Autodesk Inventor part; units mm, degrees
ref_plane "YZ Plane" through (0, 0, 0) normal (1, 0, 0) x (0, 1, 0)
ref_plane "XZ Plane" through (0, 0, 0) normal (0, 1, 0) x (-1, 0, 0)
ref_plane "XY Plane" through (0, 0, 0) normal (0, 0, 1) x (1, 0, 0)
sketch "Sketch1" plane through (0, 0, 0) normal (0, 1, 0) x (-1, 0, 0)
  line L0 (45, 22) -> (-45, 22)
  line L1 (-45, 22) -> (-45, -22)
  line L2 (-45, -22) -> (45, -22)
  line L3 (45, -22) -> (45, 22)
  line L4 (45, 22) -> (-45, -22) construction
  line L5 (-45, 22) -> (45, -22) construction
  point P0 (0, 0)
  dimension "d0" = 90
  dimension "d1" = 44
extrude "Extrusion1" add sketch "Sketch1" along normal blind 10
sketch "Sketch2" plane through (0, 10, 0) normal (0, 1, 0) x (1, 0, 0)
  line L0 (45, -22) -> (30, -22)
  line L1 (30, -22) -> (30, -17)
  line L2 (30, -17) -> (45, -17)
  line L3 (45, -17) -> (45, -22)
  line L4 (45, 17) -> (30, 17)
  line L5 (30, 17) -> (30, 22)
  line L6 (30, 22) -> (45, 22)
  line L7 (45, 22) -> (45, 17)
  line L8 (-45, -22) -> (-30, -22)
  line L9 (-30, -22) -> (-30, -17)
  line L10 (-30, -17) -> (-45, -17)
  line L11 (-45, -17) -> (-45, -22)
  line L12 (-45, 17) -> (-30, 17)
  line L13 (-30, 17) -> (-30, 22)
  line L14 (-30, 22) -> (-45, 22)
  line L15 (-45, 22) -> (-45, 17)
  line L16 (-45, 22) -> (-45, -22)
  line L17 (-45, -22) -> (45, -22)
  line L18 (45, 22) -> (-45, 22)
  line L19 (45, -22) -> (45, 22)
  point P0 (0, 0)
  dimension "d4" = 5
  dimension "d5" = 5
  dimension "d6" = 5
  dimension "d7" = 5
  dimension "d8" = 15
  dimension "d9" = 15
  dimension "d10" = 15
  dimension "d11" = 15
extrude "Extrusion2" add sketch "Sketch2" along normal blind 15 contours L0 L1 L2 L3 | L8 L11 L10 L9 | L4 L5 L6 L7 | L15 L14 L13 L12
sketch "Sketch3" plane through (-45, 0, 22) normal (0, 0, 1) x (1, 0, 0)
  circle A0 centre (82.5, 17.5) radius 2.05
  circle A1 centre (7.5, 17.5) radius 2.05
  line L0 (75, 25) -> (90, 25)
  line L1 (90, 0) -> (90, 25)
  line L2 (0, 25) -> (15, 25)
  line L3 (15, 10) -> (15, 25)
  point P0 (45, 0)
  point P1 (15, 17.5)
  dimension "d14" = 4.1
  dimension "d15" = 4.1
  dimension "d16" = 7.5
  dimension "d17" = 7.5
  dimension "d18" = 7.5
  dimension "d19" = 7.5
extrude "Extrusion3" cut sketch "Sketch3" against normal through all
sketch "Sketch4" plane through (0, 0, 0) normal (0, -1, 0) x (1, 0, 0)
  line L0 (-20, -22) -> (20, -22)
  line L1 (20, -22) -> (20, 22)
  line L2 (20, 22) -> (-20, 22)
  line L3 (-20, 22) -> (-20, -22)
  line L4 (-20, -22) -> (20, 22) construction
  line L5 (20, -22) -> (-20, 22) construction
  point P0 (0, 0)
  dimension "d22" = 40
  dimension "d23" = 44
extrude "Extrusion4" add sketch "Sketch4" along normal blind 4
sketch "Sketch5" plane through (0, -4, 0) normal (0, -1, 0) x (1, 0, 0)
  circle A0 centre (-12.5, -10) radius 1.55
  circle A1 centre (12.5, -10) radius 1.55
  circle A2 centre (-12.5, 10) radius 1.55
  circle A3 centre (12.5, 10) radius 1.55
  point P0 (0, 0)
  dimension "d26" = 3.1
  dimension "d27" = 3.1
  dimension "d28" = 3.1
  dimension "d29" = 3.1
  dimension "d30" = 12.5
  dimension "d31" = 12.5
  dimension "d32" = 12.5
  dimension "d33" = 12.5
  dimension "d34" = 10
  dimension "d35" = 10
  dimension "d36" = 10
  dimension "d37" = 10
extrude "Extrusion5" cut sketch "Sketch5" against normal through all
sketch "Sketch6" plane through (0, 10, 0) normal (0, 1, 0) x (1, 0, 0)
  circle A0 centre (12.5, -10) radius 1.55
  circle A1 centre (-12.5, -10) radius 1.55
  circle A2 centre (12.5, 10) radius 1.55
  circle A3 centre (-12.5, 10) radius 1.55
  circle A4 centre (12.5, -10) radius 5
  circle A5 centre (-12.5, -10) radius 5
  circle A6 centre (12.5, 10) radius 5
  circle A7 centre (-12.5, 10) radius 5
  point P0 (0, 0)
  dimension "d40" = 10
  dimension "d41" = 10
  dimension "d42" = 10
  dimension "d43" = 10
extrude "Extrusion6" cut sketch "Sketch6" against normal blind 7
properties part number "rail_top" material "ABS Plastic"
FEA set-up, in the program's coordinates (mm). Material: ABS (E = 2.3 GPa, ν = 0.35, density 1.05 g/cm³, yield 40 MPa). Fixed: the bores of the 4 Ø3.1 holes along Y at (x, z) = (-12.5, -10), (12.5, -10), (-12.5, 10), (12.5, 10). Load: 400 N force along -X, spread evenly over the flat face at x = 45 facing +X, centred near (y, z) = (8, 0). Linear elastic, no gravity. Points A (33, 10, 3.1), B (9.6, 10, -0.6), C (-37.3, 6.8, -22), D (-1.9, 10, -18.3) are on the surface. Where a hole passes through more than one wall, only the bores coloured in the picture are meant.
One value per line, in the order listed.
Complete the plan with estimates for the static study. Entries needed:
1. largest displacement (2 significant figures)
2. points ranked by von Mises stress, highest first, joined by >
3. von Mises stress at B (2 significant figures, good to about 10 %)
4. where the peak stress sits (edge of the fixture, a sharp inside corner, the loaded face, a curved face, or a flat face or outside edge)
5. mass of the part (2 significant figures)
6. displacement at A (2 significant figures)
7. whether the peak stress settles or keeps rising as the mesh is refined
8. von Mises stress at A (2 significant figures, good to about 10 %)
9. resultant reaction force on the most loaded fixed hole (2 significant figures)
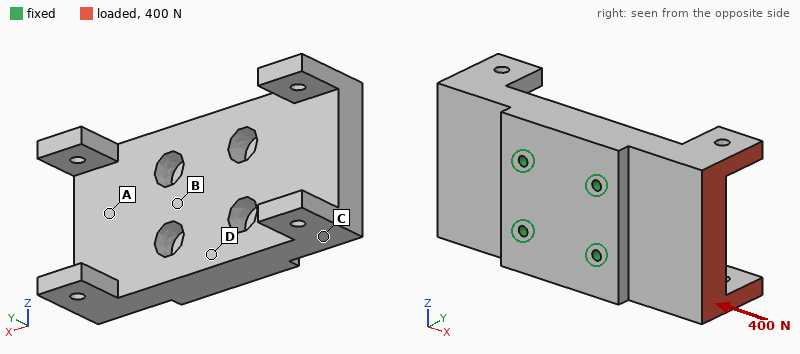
0.21 mm
B > A > D > C
2.3 MPa
edge of the fixture
51 g
0.076 mm
keeps rising
1.6 MPa
120 N
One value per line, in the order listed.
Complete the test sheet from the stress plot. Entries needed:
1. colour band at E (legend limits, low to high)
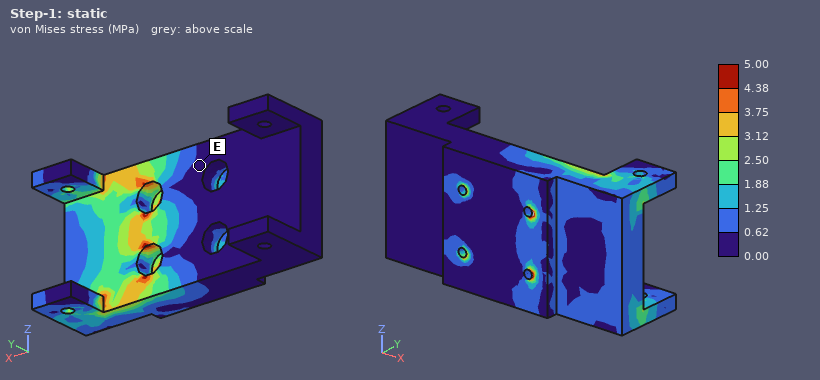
0.00 to 0.62 MPa
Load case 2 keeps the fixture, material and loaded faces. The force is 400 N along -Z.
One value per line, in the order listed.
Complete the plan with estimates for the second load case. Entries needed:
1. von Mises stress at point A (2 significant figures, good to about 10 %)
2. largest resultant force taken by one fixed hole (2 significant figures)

3.1 MPa
420 N
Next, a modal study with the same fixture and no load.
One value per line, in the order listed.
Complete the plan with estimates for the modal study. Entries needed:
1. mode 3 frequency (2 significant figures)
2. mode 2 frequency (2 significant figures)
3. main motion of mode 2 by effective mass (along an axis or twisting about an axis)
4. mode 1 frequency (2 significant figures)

2200 Hz
1600 Hz
along Y
1500 Hz
